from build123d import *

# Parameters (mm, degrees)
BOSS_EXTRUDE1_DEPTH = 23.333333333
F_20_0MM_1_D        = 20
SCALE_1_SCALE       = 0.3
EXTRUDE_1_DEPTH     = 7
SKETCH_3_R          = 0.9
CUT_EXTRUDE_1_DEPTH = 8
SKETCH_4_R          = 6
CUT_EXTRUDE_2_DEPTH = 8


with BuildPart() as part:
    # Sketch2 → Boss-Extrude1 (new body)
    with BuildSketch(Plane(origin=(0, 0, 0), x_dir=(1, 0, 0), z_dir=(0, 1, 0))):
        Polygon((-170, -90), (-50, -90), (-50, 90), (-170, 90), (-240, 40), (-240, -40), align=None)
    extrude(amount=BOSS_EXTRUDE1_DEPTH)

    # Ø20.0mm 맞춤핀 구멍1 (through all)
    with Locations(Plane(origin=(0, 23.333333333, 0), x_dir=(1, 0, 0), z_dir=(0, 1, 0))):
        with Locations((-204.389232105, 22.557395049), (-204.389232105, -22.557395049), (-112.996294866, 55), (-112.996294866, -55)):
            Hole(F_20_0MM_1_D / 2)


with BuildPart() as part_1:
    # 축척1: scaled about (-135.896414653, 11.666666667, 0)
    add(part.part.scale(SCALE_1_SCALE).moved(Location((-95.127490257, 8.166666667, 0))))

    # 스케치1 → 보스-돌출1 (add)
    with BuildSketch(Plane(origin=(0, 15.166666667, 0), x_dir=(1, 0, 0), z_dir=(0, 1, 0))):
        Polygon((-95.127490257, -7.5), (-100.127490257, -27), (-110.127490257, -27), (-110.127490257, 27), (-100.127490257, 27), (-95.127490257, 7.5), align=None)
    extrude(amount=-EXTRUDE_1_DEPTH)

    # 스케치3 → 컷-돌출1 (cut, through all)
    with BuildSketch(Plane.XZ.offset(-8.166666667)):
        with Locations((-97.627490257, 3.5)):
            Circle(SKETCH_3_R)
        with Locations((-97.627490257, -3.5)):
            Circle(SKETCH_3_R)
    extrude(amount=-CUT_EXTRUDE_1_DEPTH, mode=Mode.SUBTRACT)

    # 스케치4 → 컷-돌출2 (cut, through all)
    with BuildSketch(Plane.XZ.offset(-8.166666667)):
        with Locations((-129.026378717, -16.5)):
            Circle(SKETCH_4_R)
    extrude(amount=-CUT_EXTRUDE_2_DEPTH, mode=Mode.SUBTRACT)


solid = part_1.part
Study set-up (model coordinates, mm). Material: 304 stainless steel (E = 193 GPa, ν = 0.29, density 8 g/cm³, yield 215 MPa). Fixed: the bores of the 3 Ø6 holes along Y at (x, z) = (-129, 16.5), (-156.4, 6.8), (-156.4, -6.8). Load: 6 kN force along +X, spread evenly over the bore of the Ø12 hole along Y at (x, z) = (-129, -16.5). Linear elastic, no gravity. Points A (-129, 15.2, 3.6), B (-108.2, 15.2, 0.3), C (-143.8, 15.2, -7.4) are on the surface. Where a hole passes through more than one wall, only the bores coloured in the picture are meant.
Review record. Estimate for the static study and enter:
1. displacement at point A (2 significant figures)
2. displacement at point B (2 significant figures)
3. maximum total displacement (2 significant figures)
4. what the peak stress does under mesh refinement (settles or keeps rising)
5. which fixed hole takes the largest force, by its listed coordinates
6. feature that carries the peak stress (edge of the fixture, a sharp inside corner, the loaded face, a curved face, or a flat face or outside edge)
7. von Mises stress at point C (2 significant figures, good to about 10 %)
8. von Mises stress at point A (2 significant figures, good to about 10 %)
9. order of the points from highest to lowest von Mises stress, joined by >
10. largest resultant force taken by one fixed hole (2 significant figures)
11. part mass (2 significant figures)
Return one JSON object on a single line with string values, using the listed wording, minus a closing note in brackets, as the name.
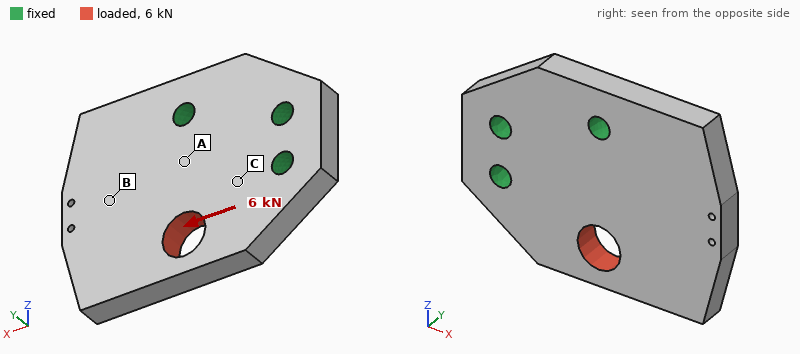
{"displacement at point A": "2.2 µm", "displacement at point B": "6.5 µm", "maximum total displacement": "13 µm", "what the peak stress does under mesh refinement": "keeps rising", "which fixed hole takes the largest force, by its listed coordinates": "(-156.4, -6.8)", "feature that carries the peak stress": "edge of the fixture", "von Mises stress at point C": "38 MPa", "von Mises stress at point A": "19 MPa", "order of the points from highest to lowest von Mises stress, joined by >": "C > A > B", "largest resultant force taken by one fixed hole": "5.0 kN", "part mass": "180 g"}
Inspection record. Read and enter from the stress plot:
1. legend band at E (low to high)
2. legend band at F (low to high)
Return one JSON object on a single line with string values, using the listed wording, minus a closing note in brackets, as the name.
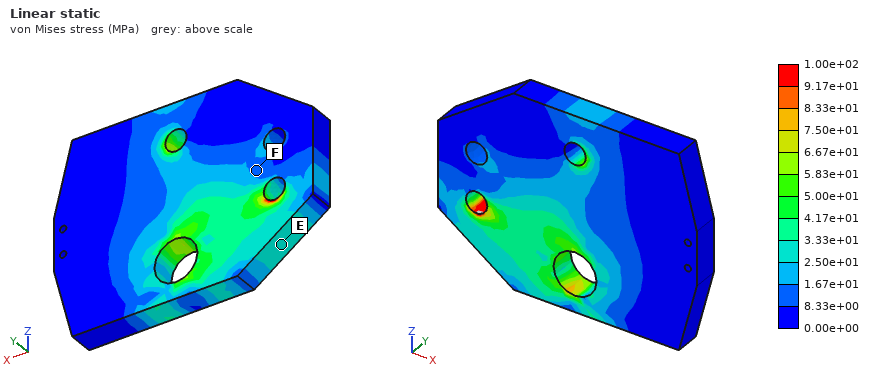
{"legend band at E": "2.50e+01 to 3.33e+01 MPa", "legend band at F": "8.33e+00 to 1.67e+01 MPa"}
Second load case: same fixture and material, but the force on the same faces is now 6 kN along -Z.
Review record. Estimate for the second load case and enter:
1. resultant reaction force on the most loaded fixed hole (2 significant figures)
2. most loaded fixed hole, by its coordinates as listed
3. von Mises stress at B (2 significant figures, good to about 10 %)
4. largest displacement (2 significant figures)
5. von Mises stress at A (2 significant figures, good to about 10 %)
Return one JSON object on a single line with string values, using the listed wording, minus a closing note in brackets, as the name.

{"resultant reaction force on the most loaded fixed hole": "4.8 kN", "most loaded fixed hole, by its coordinates as listed": "(-129, 16.5)", "von Mises stress at B": "6.9 MPa", "largest displacement": "9.9 µm", "von Mises stress at A": "35 MPa"}
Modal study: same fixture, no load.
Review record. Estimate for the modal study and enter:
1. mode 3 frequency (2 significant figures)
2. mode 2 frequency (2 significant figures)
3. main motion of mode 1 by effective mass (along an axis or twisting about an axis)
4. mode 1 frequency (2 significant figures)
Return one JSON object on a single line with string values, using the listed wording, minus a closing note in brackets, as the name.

{"mode 3 frequency": "11 kHz", "mode 2 frequency": "6300 Hz", "main motion of mode 1 by effective mass": "along Y", "mode 1 frequency": "3000 Hz"}
